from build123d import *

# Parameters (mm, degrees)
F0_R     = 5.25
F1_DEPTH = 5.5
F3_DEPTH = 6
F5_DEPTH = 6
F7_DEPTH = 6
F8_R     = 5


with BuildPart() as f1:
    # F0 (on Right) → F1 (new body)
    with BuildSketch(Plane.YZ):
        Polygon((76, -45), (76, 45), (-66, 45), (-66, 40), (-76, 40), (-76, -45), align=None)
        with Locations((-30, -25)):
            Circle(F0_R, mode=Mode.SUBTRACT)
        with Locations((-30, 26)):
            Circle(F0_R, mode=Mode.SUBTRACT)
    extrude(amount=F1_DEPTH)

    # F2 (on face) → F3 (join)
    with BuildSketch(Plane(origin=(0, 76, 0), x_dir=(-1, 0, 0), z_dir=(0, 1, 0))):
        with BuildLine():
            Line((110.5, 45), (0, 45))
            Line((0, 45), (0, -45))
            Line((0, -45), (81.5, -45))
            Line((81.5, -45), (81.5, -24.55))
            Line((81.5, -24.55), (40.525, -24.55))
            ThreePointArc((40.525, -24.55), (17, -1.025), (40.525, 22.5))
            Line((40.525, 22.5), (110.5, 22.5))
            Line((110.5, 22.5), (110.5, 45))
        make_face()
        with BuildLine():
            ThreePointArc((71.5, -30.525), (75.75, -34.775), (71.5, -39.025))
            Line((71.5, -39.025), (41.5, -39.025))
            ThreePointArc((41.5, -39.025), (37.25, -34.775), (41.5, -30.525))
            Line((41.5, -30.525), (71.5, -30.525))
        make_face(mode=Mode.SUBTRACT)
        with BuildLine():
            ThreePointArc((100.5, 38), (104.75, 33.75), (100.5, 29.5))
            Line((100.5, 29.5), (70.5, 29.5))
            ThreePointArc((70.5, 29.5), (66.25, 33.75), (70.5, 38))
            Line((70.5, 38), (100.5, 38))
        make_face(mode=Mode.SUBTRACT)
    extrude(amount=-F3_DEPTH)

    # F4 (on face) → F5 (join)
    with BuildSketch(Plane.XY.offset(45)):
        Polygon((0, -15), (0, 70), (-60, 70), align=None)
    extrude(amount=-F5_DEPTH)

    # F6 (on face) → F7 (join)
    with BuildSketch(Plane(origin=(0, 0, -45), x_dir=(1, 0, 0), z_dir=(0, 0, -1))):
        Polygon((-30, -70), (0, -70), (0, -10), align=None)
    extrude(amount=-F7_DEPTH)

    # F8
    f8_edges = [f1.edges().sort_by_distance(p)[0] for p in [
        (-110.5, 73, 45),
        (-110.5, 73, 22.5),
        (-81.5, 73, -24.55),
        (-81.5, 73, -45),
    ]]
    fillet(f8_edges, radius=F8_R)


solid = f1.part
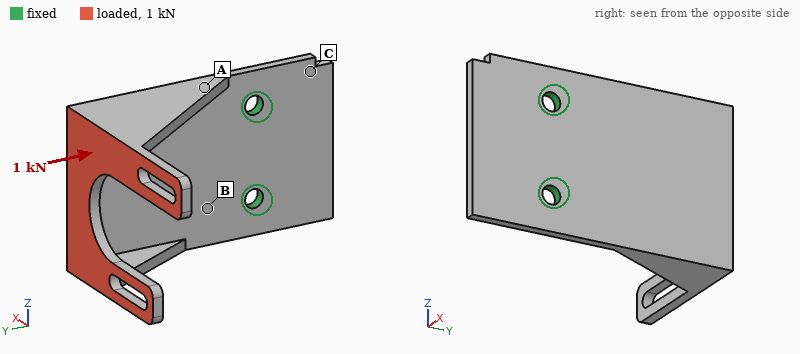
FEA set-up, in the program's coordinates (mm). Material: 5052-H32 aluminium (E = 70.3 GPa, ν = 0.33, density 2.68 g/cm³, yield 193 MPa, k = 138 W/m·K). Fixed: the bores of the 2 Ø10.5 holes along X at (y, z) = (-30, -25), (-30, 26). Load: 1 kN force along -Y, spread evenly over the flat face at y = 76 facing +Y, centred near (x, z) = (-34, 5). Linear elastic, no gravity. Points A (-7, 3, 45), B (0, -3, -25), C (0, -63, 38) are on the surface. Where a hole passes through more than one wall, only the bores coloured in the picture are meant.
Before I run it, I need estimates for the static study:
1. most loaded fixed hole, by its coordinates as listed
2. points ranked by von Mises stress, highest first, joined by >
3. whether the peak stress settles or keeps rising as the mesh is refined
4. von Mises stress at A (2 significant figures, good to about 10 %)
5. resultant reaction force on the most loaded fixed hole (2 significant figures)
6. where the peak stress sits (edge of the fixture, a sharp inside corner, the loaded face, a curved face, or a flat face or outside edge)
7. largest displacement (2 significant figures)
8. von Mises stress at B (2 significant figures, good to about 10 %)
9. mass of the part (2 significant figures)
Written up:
(-30, 26)
B > A > C
keeps rising
31 MPa
590 N
edge of the fixture
2.3 mm
55 MPa
330 g
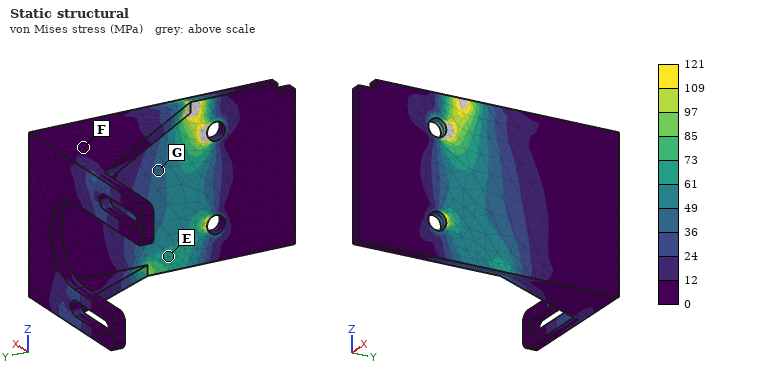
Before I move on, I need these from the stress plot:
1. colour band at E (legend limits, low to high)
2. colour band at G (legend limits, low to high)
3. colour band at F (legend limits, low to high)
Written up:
61 to 73 MPa
36 to 49 MPa
0 to 12 MPa
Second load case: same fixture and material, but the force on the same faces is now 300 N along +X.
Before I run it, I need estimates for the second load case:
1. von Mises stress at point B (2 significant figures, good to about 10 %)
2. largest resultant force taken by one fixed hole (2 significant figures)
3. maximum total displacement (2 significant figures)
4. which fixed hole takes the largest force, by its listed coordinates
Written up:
37 MPa
220 N
1.4 mm
(-30, 26)
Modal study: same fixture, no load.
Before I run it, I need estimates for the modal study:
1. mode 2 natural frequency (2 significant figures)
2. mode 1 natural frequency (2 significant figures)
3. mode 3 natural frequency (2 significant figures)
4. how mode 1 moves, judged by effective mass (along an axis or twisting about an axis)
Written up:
440 Hz
230 Hz
1300 Hz
along X
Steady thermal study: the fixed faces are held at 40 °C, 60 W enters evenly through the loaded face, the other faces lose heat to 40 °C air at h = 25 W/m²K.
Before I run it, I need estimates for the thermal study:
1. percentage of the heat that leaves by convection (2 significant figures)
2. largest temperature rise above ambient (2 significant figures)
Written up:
47 %
69 K
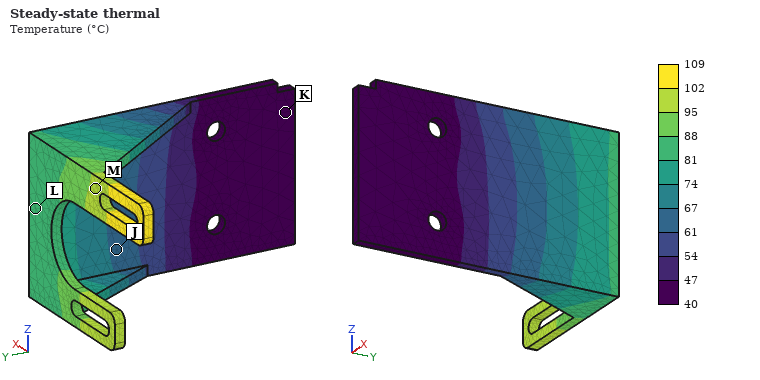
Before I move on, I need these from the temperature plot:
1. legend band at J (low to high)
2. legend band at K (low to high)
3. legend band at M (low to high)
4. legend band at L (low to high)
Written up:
61 to 67 °C
40 to 47 °C
95 to 102 °C
81 to 88 °C
